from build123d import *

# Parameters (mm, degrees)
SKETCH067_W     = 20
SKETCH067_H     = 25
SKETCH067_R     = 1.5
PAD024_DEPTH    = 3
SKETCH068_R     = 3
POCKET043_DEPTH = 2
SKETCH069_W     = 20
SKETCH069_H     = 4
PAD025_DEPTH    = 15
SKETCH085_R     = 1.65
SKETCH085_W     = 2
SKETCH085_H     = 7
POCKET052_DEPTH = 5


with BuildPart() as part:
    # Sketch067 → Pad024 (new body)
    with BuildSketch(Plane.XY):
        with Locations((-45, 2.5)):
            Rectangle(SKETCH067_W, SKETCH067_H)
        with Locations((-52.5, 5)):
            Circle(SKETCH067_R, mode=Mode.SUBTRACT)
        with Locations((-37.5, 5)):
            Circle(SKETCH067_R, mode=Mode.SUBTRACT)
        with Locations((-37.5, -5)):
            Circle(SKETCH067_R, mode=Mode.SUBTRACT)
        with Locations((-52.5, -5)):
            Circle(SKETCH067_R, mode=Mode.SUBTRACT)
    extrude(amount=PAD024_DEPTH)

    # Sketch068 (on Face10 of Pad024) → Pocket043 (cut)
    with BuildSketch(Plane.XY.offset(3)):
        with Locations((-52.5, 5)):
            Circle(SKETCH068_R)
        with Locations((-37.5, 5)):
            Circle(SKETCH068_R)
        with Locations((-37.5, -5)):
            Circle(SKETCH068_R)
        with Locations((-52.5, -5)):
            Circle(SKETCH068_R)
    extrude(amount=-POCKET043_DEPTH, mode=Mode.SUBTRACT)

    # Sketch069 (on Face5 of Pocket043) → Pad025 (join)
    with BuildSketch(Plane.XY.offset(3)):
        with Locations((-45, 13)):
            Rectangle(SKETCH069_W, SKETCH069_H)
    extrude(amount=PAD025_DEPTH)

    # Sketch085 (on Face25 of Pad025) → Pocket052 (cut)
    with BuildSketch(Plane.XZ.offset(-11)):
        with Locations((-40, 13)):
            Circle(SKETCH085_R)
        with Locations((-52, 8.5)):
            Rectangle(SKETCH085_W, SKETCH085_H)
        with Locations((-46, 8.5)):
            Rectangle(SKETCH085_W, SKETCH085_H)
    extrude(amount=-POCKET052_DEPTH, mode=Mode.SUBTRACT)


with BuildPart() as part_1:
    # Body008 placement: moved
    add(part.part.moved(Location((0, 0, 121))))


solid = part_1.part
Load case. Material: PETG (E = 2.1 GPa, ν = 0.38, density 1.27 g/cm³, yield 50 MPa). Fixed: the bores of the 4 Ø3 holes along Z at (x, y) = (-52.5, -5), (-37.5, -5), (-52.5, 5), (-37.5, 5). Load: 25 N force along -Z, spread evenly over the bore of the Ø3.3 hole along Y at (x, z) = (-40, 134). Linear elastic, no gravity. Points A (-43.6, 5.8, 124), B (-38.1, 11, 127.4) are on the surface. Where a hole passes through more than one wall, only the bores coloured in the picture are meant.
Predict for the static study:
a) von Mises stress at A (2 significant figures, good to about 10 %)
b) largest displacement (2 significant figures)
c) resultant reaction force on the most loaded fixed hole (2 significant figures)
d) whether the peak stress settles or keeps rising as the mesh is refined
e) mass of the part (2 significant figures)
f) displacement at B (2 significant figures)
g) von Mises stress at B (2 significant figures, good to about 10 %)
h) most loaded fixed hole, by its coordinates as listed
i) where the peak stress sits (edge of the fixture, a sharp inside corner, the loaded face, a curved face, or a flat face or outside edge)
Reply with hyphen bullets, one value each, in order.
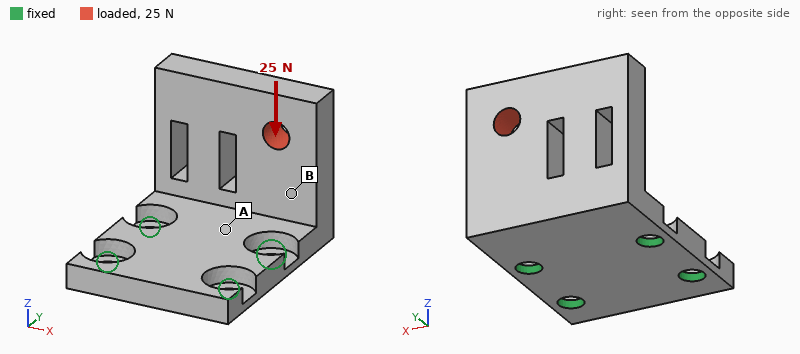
- 6.7 MPa
- 0.39 mm
- 33 N
- keeps rising
- 2.9 g
- 0.16 mm
- 1.5 MPa
- (-37.5, 5)
- edge of the fixture
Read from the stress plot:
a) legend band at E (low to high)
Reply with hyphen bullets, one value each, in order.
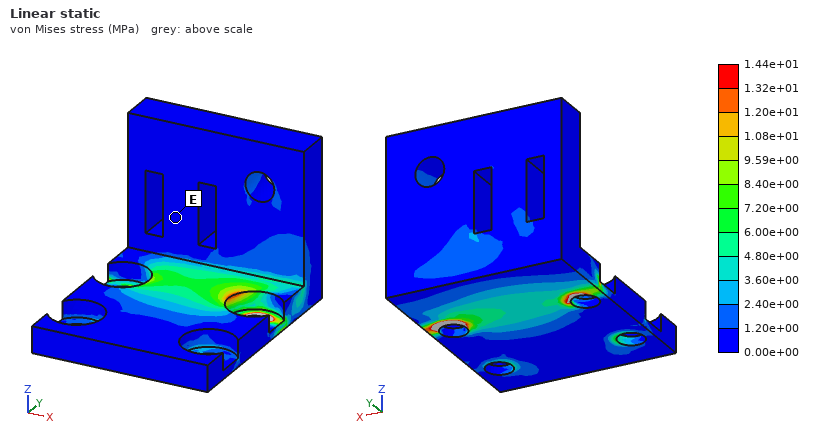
- 0.00e+00 to 1.20e+00 MPa
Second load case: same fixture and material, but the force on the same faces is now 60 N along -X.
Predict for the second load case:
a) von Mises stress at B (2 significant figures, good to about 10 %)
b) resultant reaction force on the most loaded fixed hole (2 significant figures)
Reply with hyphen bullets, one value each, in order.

- 5.7 MPa
- 66 N
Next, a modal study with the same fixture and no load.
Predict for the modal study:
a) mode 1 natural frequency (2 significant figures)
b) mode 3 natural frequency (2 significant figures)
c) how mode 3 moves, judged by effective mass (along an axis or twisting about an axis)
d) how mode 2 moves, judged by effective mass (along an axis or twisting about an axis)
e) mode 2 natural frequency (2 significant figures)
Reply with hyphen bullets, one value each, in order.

- 940 Hz
- 3700 Hz
- along Z
- along X
- 2100 Hz
